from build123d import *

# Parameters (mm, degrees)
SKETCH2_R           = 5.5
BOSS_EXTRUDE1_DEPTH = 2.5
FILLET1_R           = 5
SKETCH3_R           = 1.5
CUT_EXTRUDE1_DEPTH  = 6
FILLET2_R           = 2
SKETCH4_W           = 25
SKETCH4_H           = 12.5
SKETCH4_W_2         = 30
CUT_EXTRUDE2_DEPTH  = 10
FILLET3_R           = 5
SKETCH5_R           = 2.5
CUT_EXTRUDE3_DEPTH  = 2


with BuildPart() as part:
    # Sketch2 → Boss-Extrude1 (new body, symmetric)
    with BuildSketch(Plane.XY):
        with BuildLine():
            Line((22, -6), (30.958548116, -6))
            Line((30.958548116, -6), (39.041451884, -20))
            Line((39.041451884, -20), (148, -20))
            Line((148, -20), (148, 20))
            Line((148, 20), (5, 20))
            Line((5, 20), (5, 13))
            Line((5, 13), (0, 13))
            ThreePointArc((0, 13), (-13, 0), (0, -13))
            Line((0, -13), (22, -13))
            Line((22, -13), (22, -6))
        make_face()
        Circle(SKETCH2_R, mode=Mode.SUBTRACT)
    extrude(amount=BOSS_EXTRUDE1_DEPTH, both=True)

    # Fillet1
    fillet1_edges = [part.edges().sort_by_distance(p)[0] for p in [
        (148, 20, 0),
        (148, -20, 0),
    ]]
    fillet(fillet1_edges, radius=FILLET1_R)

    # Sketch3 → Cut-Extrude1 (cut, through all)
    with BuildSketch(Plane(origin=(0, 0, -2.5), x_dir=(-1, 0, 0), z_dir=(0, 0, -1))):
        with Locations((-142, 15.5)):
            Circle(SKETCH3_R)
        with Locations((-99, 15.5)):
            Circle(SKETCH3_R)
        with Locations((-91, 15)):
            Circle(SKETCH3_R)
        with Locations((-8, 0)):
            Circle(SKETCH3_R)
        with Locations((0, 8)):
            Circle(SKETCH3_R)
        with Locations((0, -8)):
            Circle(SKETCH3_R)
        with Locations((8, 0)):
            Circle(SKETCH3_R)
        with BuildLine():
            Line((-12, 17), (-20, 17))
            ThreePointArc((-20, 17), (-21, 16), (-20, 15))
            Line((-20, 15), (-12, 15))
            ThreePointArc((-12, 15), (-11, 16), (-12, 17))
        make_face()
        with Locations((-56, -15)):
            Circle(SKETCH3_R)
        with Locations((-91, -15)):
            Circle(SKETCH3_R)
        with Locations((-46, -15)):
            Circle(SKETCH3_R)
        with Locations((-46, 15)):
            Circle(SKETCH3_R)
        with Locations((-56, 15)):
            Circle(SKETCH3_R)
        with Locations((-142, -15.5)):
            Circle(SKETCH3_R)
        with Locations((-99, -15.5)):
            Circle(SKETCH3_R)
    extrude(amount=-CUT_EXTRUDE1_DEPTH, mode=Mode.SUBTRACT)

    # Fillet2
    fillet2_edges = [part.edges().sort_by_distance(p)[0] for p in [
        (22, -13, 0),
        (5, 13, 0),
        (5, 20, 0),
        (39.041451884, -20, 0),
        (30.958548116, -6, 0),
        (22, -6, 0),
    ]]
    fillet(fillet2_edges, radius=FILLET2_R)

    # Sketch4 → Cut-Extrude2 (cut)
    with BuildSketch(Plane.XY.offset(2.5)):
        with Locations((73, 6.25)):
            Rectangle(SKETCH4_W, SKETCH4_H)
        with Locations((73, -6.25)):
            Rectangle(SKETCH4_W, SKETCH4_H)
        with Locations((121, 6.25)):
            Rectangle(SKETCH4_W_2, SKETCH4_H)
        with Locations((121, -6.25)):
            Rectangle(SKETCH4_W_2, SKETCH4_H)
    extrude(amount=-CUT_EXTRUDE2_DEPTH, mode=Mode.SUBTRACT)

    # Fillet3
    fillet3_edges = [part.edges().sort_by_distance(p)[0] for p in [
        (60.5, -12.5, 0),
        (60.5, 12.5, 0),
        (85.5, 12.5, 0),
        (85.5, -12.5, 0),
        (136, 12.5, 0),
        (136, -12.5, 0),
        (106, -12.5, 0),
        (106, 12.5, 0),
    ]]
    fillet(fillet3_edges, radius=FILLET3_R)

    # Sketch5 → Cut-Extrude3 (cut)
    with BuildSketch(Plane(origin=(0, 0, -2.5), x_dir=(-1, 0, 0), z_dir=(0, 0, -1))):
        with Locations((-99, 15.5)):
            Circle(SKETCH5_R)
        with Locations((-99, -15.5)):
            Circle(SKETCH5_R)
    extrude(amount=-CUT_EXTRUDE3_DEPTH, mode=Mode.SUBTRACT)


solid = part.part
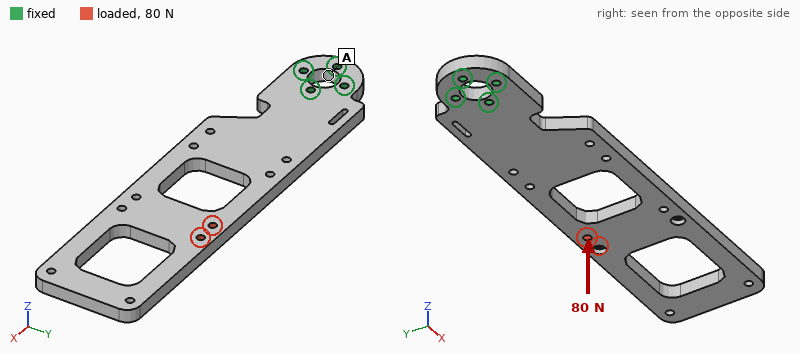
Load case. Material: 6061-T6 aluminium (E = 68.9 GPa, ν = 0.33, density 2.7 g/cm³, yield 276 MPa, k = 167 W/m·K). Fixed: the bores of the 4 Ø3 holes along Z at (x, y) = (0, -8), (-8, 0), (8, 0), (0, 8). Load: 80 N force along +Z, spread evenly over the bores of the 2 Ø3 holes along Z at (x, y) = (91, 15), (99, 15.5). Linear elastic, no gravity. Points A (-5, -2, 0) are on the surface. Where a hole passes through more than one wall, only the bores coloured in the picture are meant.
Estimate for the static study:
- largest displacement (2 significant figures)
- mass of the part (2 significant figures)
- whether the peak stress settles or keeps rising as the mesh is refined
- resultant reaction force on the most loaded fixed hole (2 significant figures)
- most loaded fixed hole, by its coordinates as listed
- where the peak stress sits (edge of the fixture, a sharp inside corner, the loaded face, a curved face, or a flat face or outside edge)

1.9 mm
57 g
keeps rising
460 N
(8, 0)
edge of the fixture
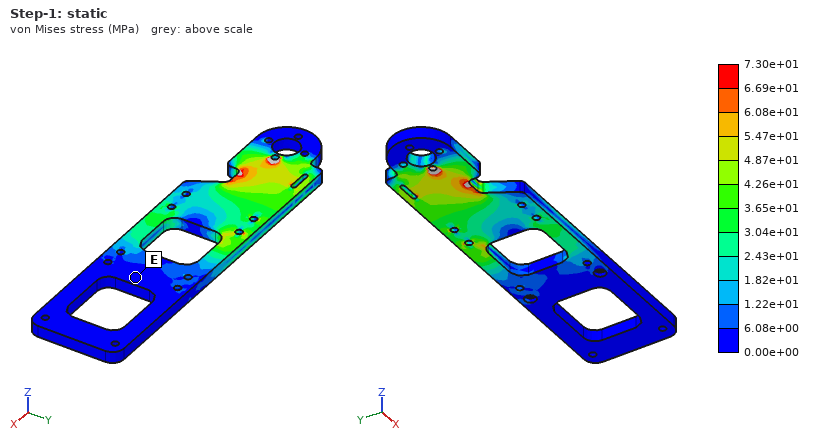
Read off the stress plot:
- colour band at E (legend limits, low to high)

0.00e+00 to 6.08e+00 MPa
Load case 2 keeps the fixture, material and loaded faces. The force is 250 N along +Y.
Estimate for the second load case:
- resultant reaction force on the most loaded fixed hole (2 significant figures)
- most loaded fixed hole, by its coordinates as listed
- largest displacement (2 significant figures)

1.1 kN
(0, 8)
0.25 mm
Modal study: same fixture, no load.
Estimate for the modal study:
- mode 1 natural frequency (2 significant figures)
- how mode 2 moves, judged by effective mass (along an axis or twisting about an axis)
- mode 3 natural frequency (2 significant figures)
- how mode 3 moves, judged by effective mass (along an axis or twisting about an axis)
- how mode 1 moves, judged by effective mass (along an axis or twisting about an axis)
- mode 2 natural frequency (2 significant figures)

200 Hz
along Y
1100 Hz
along Z
along Z
980 Hz
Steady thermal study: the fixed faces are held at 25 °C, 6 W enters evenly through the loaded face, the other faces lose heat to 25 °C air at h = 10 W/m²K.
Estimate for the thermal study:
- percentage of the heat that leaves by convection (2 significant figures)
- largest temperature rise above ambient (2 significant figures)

26 %
25 K
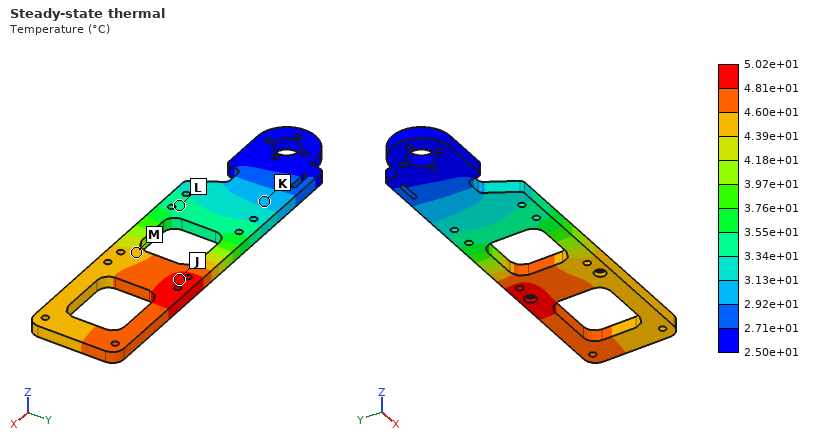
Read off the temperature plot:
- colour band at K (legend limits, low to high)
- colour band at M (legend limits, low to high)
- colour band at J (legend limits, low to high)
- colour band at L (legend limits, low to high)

2.92e+01 to 3.13e+01 °C
4.39e+01 to 4.60e+01 °C
4.81e+01 to 5.02e+01 °C
3.34e+01 to 3.55e+01 °C
